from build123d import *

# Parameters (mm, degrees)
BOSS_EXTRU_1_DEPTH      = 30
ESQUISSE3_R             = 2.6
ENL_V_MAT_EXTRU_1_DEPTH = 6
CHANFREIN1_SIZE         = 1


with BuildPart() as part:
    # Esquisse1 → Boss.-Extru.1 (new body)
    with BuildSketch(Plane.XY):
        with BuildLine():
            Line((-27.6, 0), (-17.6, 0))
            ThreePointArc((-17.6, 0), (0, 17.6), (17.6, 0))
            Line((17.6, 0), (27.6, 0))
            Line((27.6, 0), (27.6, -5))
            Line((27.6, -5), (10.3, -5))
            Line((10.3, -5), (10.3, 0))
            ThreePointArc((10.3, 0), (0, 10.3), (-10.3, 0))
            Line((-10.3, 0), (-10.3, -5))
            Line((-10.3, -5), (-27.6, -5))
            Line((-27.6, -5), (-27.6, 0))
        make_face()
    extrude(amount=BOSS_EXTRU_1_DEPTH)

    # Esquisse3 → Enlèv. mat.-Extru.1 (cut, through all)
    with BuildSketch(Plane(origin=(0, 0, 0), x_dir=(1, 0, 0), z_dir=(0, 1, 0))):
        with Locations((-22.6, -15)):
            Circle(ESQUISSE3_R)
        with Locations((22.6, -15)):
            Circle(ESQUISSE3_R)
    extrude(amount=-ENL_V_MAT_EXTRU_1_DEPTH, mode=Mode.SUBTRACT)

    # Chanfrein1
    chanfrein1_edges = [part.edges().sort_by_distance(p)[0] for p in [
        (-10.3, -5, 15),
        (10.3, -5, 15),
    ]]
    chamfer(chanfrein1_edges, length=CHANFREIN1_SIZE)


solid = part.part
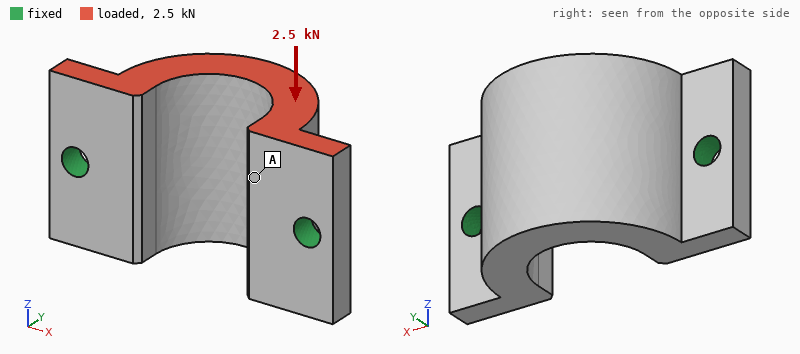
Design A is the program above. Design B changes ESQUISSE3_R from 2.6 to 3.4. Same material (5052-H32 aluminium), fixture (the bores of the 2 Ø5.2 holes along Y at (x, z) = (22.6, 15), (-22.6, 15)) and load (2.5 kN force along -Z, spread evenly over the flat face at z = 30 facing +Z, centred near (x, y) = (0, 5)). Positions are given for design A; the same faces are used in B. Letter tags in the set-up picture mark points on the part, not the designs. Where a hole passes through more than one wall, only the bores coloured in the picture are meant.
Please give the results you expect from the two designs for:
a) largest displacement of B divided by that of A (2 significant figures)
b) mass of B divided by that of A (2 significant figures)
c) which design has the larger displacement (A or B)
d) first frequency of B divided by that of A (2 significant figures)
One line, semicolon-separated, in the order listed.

0.72; 0.99; A; 1.2
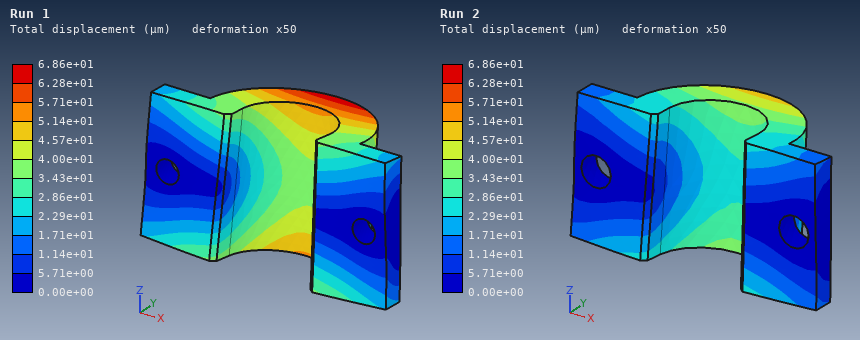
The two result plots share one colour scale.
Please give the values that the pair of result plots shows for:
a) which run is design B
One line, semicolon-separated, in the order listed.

Run 2
